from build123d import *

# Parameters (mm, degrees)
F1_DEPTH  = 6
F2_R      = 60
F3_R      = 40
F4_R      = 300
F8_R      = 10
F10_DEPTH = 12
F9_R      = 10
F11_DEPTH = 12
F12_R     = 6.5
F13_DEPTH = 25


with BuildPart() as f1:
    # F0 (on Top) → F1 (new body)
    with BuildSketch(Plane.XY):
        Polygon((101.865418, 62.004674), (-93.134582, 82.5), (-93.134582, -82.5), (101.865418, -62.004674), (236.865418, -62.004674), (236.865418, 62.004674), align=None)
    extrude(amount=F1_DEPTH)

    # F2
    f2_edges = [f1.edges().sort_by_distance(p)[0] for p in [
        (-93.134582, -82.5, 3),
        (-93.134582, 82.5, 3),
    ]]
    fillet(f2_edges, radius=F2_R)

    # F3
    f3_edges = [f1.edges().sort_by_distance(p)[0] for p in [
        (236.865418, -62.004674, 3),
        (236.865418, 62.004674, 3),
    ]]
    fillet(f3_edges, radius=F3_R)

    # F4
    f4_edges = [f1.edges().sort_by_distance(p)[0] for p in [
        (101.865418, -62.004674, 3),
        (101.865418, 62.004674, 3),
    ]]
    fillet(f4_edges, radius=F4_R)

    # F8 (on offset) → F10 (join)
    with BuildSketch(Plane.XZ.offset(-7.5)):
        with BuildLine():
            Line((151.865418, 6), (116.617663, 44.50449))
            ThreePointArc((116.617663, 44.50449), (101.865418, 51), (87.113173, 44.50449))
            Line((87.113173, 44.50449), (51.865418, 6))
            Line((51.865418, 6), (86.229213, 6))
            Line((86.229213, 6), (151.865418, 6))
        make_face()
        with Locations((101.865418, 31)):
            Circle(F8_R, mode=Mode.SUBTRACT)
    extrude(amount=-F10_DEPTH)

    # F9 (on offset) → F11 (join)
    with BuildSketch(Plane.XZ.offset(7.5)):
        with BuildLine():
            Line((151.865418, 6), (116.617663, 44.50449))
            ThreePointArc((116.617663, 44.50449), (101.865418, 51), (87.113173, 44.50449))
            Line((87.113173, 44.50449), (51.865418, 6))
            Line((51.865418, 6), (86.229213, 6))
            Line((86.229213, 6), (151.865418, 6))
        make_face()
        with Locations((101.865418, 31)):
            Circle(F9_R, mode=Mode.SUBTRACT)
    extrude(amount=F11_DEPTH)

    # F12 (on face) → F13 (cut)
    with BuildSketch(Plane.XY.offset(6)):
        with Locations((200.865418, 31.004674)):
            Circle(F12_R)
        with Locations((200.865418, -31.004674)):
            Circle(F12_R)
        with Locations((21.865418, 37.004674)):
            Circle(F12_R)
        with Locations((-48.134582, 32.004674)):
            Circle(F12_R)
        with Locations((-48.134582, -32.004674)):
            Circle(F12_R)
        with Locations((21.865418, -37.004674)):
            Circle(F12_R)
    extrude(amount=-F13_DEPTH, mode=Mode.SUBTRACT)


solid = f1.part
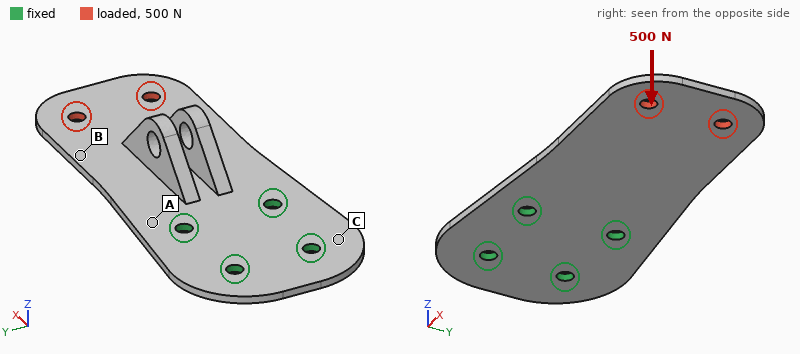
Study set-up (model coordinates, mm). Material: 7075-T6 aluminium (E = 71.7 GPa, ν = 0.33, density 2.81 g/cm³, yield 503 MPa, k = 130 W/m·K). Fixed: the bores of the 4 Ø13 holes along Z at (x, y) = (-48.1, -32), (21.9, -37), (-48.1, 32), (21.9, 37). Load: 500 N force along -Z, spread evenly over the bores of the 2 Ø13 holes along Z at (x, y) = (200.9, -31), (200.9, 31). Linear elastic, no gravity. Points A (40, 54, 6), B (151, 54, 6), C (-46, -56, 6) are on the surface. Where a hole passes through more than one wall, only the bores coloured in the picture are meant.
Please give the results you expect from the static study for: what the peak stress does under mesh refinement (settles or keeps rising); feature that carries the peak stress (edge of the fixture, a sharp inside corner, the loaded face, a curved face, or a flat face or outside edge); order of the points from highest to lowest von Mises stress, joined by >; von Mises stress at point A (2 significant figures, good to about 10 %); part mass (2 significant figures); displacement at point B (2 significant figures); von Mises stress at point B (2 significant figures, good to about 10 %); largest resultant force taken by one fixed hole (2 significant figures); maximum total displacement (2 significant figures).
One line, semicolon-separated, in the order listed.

keeps rising; edge of the fixture; A > B > C; 81 MPa; 860 g; 1.9 mm; 18 MPa; 370 N; 3.8 mm
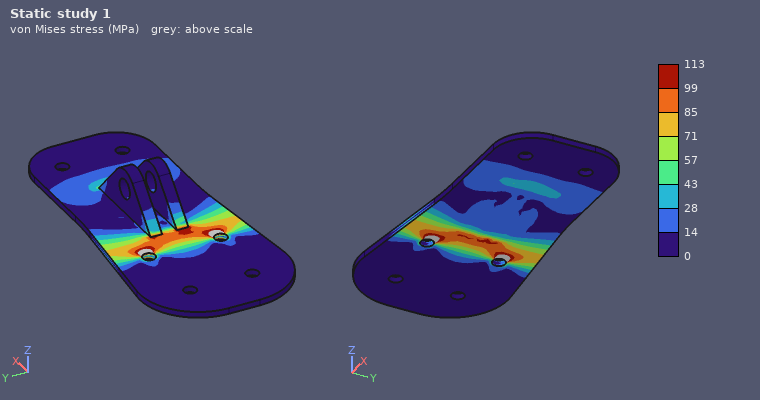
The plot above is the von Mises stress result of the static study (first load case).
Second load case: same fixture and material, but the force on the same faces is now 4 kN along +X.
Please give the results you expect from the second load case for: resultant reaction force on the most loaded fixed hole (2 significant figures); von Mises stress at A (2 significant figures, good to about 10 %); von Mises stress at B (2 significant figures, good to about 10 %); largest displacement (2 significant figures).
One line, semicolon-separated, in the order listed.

1.7 kN; 3.8 MPa; 4.3 MPa; 51 µm
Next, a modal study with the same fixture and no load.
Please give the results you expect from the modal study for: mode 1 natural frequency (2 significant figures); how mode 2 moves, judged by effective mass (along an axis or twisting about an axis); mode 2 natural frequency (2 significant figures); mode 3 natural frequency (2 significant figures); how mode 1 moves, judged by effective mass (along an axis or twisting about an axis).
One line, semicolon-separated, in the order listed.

140 Hz; twisting about X; 590 Hz; 870 Hz; along Z
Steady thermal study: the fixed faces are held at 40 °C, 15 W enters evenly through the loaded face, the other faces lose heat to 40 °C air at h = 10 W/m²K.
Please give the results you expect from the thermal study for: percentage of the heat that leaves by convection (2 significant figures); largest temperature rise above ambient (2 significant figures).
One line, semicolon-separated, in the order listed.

39 %; 19 K
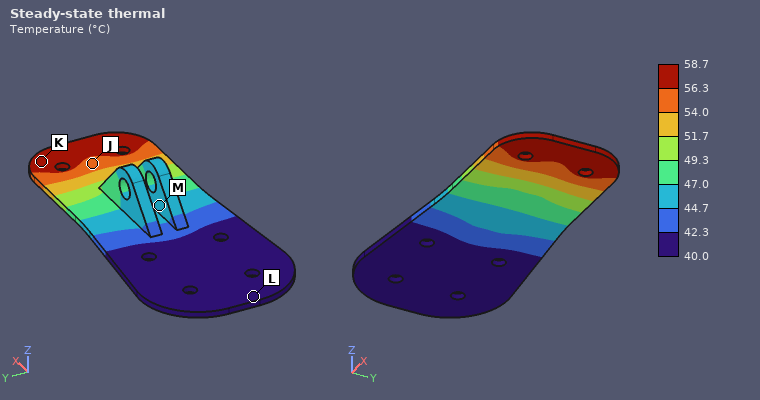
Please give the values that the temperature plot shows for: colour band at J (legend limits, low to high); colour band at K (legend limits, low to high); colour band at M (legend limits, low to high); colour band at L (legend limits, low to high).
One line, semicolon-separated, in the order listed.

54.0 to 56.3 °C; 56.3 to 58.7 °C; 44.7 to 47.0 °C; 40.0 to 42.3 °C
